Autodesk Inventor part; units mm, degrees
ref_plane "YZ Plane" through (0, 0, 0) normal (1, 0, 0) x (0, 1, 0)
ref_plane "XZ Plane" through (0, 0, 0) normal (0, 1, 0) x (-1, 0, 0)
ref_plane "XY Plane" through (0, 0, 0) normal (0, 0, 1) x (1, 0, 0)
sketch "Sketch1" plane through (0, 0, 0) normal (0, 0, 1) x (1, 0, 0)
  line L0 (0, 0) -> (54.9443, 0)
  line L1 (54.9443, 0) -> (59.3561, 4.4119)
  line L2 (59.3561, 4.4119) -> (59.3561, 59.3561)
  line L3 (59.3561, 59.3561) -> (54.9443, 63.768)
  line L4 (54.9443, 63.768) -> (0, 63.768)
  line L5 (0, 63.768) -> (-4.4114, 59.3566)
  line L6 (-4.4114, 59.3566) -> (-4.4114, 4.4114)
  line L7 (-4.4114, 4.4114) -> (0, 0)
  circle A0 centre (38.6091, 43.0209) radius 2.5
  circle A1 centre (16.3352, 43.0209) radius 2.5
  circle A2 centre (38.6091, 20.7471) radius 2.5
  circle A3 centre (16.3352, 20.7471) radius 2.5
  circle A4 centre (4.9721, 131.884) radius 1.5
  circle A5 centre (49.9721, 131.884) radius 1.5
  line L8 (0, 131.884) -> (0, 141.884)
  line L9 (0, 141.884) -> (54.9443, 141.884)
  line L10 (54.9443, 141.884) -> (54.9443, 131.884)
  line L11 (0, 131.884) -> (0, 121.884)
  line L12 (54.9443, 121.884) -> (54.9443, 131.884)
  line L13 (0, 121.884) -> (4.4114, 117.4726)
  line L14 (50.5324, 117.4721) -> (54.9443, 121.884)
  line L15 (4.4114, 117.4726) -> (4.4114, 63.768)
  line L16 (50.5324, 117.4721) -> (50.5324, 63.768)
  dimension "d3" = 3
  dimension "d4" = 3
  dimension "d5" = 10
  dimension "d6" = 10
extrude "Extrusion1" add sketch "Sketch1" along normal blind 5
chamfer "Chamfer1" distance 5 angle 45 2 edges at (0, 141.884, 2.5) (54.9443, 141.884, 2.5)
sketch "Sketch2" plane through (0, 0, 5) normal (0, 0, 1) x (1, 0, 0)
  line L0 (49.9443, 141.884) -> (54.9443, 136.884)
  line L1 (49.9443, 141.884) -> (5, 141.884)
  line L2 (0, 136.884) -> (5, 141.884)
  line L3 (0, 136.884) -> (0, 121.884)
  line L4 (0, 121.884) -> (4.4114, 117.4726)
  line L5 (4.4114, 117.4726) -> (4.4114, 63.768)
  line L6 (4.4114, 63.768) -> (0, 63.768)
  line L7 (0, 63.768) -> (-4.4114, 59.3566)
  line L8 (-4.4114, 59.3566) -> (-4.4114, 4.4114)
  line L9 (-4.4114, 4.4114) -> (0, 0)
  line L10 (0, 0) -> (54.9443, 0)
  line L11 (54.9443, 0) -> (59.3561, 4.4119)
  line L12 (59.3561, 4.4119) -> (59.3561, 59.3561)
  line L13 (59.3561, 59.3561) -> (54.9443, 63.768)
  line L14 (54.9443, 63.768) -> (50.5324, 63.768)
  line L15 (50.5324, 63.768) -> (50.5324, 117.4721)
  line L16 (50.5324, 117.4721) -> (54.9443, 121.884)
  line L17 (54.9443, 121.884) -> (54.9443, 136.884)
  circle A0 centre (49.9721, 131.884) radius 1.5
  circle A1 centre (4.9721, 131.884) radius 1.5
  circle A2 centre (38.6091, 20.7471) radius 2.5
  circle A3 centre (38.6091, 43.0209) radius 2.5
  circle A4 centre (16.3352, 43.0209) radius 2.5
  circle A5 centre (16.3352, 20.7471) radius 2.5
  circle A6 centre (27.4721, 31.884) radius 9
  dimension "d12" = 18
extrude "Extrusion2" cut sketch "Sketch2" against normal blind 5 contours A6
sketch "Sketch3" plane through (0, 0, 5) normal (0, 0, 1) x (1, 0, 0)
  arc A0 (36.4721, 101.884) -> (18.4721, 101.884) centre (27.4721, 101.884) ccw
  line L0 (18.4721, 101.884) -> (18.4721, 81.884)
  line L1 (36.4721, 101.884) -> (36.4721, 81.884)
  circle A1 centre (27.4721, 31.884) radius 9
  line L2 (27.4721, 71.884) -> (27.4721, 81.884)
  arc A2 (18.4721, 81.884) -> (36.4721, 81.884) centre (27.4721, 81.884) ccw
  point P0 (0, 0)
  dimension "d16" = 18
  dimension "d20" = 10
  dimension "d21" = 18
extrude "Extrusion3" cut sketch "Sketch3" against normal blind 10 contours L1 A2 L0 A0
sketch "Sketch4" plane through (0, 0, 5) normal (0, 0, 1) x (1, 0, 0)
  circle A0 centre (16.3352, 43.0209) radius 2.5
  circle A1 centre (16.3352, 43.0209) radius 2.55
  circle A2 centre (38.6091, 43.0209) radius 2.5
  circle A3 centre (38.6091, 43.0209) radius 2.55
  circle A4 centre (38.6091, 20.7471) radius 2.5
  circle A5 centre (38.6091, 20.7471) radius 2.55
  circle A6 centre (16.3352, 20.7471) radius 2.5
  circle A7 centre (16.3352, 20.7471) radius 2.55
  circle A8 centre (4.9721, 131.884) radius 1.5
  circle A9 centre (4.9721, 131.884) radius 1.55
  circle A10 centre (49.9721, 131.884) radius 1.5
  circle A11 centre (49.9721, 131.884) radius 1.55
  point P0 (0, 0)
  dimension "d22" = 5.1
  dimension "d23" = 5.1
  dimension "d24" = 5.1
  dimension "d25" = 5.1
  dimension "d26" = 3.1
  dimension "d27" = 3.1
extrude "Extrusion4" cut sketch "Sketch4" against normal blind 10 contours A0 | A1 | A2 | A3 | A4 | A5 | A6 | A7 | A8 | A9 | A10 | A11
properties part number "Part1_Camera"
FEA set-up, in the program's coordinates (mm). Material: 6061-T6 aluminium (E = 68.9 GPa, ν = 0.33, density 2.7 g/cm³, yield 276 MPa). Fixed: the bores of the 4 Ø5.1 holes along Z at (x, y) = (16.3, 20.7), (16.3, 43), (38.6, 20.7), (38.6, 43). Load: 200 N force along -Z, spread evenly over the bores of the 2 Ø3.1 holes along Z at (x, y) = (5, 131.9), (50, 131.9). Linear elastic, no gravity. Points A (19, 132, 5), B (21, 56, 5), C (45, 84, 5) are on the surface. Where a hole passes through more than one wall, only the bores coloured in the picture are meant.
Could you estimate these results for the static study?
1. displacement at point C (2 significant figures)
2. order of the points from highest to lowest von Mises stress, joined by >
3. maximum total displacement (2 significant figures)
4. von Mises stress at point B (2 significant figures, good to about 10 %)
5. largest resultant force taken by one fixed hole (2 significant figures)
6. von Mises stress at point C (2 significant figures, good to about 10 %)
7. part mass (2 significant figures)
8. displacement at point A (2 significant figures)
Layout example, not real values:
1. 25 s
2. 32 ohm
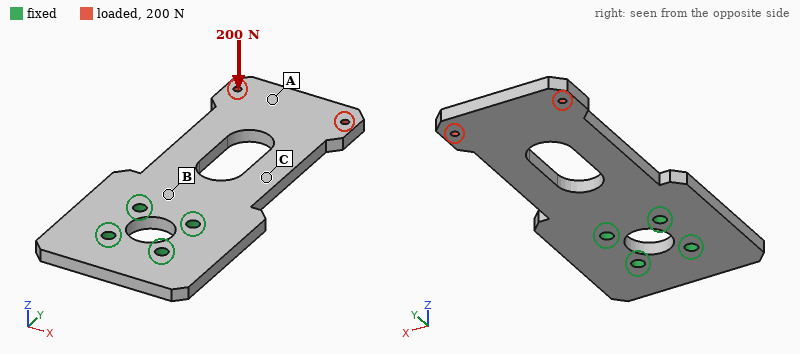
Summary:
1. 0.34 mm
2. C > B > A
3. 1.8 mm
4. 60 MPa
5. 200 N
6. 80 MPa
7. 92 g
8. 1.5 mm
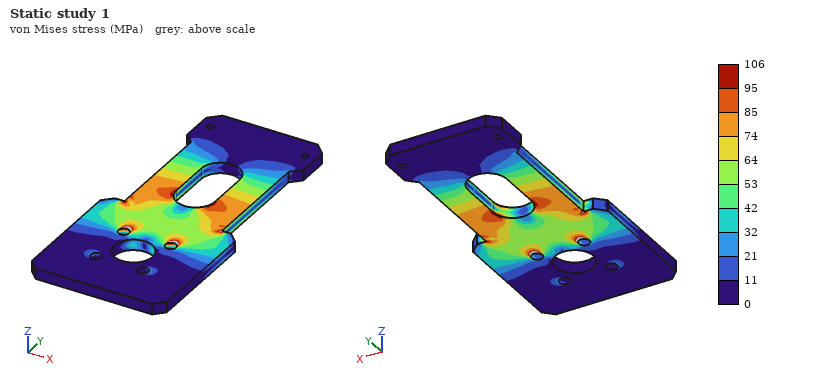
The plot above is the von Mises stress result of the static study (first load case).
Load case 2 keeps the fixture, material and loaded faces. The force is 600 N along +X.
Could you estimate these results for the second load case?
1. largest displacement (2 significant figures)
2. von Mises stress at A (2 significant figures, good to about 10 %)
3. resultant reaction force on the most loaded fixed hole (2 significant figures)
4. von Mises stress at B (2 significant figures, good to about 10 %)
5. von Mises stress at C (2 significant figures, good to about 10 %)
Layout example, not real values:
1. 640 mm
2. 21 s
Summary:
1. 94 µm
2. 4.5 MPa
3. 1.3 kN
4. 7.1 MPa
5. 17 MPa
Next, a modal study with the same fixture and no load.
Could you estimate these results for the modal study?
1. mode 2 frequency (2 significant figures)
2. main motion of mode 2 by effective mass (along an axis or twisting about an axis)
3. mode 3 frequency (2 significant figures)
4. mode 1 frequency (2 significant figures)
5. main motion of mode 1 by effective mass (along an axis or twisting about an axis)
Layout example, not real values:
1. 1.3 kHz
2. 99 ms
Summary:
1. 1500 Hz
2. twisting about Y
3. 2600 Hz
4. 410 Hz
5. along Z
